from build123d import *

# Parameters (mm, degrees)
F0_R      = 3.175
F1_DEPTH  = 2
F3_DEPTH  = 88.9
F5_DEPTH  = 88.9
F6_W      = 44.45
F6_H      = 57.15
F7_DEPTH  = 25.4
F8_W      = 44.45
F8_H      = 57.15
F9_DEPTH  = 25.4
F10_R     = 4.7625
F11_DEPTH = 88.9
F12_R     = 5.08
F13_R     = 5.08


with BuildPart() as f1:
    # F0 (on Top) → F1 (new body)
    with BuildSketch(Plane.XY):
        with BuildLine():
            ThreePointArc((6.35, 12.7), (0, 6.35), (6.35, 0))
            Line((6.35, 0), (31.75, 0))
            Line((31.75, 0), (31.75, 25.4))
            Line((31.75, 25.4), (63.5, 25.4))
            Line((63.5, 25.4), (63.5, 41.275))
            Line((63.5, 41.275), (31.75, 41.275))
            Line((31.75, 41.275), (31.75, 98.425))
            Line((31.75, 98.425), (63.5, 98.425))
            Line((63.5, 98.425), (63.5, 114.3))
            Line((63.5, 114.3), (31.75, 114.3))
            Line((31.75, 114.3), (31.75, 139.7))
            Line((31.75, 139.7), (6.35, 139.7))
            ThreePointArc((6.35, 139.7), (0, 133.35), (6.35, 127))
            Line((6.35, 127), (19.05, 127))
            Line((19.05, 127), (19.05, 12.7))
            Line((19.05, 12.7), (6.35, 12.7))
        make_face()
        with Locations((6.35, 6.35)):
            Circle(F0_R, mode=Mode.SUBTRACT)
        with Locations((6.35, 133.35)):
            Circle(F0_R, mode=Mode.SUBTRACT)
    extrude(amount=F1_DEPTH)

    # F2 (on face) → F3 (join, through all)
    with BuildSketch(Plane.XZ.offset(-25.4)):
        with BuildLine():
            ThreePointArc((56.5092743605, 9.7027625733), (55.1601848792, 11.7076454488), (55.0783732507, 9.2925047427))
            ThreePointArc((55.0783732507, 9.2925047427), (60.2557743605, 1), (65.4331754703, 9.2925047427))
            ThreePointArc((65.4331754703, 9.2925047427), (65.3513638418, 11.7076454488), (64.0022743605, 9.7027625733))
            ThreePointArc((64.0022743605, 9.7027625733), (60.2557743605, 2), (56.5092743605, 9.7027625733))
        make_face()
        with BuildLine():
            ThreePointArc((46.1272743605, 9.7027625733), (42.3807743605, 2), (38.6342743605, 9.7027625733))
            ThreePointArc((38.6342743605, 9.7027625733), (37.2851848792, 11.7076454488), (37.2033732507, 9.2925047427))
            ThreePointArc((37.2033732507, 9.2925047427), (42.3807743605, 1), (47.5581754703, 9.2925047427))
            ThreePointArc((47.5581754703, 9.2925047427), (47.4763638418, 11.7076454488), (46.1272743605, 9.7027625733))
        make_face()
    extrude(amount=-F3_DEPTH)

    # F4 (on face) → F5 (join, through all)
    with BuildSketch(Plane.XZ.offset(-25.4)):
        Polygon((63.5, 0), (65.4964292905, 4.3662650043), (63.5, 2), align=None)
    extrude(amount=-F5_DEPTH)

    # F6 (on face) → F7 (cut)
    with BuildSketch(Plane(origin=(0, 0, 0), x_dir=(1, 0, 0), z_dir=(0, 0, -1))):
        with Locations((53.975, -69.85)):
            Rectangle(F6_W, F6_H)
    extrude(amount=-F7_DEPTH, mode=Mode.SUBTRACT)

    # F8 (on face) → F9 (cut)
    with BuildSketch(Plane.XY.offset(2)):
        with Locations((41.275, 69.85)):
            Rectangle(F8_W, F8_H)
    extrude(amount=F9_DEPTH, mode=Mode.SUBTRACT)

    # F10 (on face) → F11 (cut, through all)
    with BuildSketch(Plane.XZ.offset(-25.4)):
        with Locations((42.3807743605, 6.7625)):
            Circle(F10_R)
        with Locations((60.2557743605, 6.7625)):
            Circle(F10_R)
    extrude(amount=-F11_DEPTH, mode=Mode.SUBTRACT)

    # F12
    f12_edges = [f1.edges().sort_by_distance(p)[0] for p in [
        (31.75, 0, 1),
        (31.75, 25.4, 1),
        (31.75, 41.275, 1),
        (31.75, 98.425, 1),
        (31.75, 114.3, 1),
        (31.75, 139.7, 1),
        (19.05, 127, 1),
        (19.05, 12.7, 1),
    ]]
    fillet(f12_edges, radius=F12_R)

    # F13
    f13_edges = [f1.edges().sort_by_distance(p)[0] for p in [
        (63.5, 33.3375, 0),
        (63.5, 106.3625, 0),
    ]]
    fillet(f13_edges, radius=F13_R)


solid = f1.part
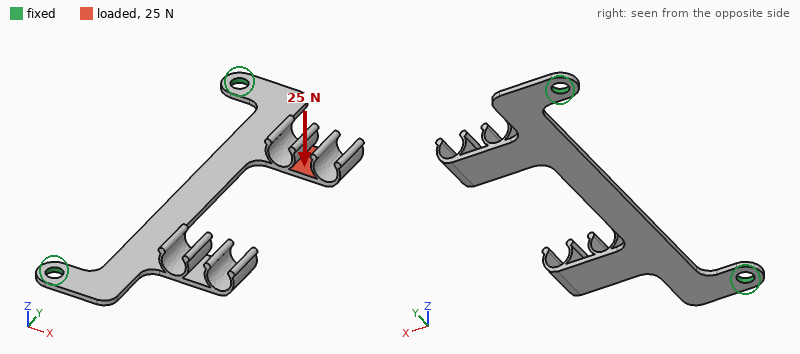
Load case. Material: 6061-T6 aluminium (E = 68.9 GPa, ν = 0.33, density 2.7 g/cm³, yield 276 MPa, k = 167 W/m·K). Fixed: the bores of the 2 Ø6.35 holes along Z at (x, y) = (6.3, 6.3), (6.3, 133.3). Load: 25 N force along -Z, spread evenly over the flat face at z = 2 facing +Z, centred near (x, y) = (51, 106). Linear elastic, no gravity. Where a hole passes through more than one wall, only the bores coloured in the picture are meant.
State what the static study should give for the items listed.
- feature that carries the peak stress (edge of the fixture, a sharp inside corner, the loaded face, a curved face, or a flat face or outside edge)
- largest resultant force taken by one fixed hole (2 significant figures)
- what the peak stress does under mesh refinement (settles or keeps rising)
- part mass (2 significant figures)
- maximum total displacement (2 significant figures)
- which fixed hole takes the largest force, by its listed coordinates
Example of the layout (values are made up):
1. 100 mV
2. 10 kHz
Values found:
1. edge of the fixture
2. 21 N
3. keeps rising
4. 22 g
5. 1.7 mm
6. (6.3, 133.3)
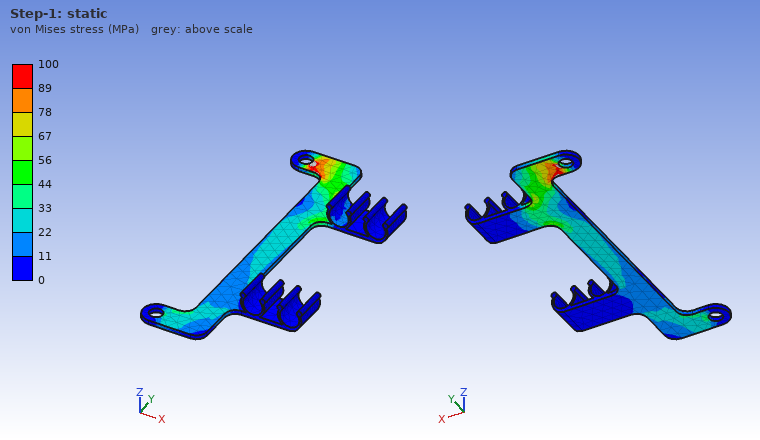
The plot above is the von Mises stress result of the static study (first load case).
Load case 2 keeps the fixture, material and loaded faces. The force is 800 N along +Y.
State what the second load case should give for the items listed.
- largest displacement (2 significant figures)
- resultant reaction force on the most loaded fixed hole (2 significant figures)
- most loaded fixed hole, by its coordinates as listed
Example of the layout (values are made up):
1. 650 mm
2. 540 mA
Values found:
1. 0.89 mm
2. 680 N
3. (6.3, 6.3)
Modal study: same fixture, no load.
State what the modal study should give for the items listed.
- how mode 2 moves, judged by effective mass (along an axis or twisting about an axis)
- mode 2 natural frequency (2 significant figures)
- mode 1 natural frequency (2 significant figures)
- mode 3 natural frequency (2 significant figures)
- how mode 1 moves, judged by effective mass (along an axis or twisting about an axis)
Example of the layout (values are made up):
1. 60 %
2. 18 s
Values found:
1. twisting about X
2. 420 Hz
3. 270 Hz
4. 660 Hz
5. along Z
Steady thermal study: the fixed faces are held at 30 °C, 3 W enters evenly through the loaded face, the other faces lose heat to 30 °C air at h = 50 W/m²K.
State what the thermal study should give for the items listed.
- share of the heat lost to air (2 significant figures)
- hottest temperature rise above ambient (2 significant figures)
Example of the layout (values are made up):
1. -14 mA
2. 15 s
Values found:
1. 70 %
2. 13 K
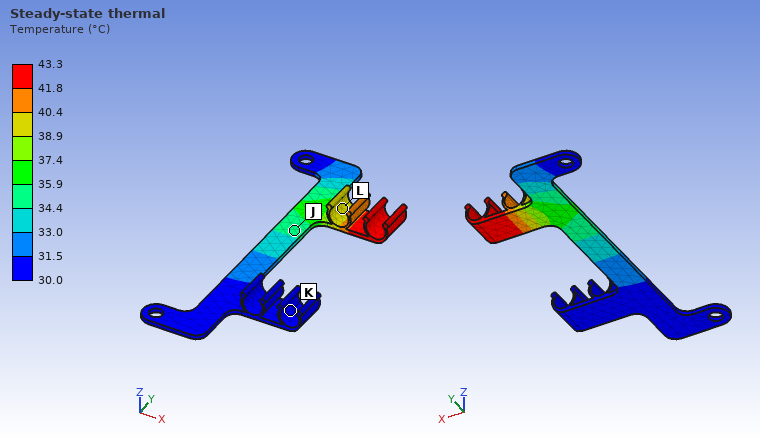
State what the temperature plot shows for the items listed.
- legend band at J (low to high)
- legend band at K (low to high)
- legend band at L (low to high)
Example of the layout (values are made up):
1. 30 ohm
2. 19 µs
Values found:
1. 34.4 to 35.9 °C
2. 30.0 to 31.5 °C
3. 38.9 to 40.4 °C
